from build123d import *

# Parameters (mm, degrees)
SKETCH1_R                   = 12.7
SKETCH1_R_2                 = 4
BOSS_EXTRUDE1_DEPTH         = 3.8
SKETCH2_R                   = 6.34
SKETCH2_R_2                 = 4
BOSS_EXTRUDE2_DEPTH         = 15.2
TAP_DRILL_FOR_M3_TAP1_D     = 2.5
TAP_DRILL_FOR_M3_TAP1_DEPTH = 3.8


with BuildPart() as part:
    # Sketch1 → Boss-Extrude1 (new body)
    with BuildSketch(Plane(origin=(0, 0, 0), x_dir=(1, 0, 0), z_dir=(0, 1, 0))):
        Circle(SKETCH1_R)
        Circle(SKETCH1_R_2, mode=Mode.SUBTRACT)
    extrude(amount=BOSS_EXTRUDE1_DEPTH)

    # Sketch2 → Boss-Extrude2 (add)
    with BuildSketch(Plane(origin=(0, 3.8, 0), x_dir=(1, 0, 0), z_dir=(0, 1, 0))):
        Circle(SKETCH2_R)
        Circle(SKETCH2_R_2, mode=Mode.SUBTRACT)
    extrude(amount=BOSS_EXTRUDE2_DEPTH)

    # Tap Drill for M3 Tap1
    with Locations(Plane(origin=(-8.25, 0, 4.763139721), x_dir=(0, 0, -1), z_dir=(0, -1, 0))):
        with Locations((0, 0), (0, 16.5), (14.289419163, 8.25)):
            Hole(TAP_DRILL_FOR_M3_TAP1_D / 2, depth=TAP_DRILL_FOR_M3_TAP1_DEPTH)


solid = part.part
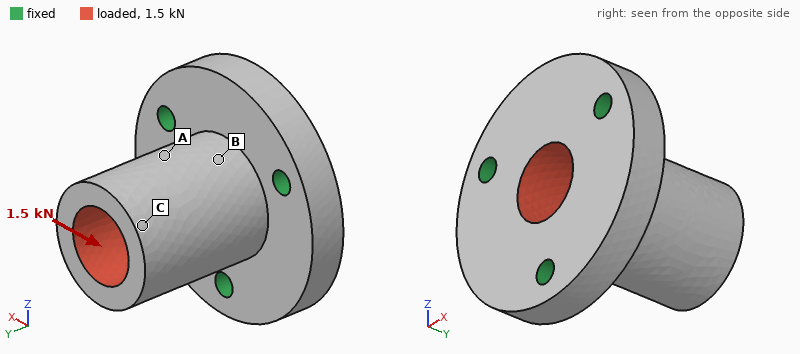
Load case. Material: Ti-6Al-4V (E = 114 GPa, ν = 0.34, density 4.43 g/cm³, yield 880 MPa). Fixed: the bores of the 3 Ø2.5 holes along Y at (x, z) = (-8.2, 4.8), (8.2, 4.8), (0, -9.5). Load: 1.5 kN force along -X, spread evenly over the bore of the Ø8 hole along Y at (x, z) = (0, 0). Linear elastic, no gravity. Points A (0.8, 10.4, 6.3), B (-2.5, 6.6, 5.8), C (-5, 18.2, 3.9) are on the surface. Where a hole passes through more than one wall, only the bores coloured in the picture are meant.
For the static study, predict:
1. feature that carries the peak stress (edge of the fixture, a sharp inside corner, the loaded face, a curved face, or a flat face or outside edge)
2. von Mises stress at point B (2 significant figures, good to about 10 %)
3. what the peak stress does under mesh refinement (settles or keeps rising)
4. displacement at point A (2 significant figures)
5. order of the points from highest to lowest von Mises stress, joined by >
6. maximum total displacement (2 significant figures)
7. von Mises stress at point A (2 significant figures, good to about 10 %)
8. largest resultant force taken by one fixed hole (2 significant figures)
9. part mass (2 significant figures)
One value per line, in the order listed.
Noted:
edge of the fixture
35 MPa
keeps rising
9.6 µm
B > A > C
21 µm
25 MPa
860 N
13 g
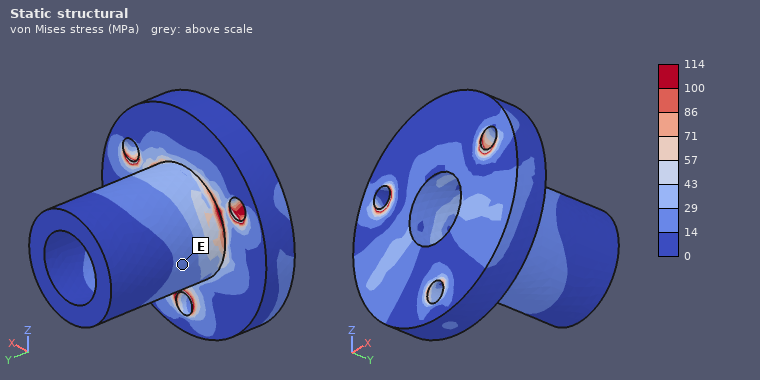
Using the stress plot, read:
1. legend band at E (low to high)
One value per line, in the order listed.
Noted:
14 to 29 MPa
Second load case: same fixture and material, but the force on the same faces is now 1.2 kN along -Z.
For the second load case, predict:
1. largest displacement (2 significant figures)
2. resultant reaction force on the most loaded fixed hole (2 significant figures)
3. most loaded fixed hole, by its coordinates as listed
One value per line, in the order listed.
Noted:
17 µm
760 N
(0, -9.5)
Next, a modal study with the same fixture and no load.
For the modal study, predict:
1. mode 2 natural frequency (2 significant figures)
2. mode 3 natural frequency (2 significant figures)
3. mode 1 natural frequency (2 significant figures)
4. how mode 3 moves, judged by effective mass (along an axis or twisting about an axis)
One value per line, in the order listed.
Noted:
19 kHz
37 kHz
19 kHz
along Y
